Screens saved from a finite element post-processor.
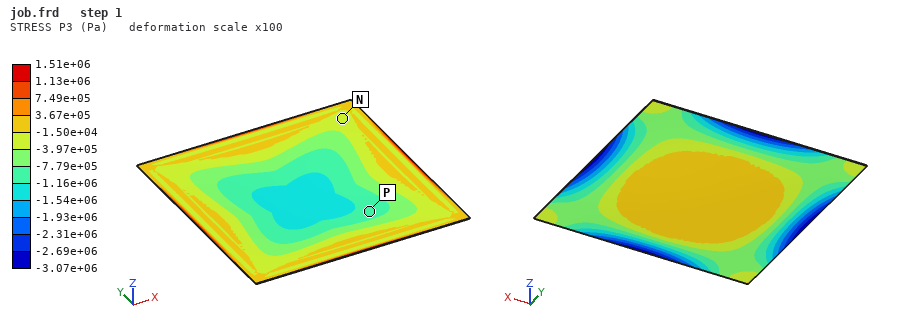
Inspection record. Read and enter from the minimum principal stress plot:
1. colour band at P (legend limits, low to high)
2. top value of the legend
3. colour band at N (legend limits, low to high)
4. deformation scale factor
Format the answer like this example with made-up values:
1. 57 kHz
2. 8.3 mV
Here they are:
1. -1.16e+06 to -7.79e+05 Pa
2. 1.51e+06 Pa
3. -3.97e+05 to -1.50e+04 Pa
4. 100
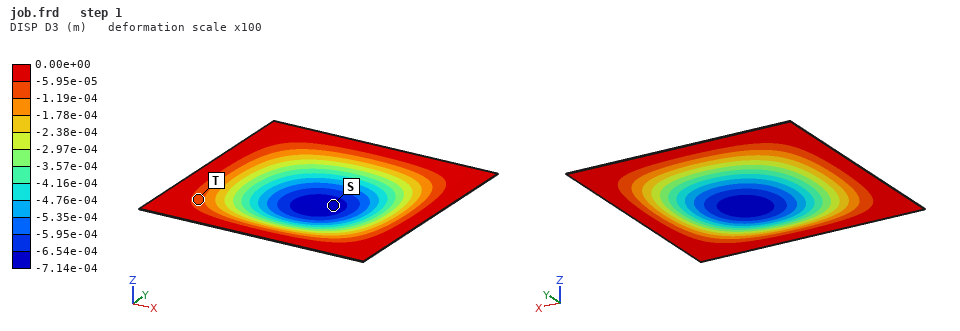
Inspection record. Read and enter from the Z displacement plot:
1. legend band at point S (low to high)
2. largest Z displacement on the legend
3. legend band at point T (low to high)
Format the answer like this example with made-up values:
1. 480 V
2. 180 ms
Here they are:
1. -7.14e-04 to -6.54e-04 m
2. 0.00e+00 m
3. -1.19e-04 to -5.95e-05 m
